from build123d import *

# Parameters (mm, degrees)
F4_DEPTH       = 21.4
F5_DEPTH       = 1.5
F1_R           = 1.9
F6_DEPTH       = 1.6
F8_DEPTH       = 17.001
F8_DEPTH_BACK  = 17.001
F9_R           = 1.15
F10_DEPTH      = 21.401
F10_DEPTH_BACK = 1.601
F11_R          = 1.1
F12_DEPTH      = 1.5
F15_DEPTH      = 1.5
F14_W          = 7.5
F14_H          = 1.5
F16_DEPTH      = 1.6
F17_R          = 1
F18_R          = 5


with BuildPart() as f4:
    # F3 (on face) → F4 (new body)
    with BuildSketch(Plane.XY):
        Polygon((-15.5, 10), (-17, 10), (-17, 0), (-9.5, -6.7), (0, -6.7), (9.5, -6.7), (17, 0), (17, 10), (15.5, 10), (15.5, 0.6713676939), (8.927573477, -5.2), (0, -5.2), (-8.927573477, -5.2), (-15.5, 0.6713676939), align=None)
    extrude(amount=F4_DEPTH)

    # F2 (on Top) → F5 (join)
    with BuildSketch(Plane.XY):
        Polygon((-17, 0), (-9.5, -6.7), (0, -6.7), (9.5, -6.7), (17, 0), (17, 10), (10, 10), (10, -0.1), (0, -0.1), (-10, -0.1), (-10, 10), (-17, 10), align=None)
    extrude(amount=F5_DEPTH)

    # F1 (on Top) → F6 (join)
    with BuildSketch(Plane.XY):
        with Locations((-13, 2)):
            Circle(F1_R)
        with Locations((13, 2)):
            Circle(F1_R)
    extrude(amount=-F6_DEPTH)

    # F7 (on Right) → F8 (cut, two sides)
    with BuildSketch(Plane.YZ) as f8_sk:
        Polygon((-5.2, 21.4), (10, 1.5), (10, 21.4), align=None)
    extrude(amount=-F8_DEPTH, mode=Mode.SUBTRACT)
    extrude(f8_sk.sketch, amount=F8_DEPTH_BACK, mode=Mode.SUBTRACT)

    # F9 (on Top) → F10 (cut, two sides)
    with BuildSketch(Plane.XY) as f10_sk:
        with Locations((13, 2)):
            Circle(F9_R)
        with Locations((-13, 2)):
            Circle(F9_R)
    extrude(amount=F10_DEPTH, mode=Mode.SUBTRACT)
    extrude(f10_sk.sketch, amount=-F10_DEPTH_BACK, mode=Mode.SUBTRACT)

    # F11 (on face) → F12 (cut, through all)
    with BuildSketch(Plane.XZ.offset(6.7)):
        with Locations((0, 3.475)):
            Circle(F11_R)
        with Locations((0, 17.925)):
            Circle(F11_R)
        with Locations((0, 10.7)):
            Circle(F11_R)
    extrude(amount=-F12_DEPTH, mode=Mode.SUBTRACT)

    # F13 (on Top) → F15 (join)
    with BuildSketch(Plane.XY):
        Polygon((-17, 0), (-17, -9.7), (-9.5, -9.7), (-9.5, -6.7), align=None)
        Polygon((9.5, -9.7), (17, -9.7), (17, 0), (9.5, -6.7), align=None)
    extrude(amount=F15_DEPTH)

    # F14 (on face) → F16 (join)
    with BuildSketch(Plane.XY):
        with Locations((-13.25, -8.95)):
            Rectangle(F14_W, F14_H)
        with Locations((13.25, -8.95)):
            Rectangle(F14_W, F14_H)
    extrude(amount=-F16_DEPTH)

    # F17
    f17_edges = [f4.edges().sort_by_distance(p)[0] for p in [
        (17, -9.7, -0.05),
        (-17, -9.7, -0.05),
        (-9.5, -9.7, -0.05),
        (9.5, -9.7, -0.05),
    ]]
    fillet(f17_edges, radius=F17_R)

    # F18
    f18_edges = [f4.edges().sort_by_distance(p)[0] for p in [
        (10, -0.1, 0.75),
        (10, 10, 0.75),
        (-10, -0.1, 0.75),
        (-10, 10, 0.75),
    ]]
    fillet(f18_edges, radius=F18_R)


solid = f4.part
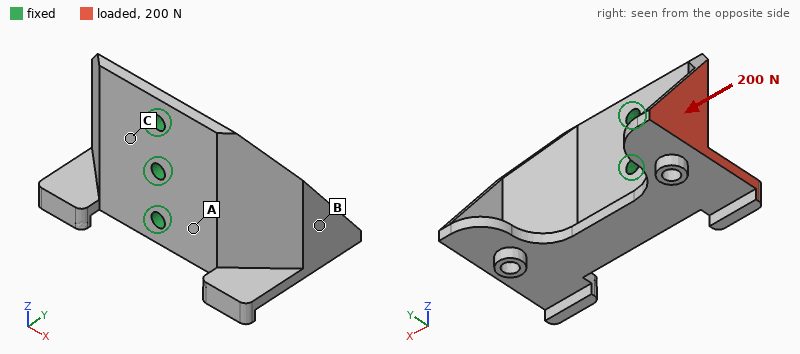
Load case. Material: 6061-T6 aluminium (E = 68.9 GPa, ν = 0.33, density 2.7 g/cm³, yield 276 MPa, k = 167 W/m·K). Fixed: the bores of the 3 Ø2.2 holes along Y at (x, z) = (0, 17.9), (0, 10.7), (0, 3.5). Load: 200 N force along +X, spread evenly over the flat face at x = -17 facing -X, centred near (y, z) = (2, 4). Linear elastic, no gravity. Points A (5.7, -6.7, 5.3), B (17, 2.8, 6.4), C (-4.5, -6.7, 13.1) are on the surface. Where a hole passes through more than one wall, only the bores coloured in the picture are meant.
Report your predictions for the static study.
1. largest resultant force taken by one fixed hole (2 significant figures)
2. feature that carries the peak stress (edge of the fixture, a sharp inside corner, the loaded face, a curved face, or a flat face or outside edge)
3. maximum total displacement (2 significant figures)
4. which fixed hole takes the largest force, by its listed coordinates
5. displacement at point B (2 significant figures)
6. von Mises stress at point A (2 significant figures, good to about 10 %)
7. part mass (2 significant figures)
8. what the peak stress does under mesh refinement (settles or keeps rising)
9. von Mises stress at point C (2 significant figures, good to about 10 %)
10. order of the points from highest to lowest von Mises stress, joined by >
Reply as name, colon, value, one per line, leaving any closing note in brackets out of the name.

largest resultant force taken by one fixed hole: 170 N
feature that carries the peak stress: edge of the fixture
maximum total displacement: 0.22 mm
which fixed hole takes the largest force, by its listed coordinates: (0, 3.5)
displacement at point B: 0.099 mm
von Mises stress at point A: 30 MPa
part mass: 5.0 g
what the peak stress does under mesh refinement: keeps rising
von Mises stress at point C: 51 MPa
order of the points from highest to lowest von Mises stress, joined by >: C > A > B
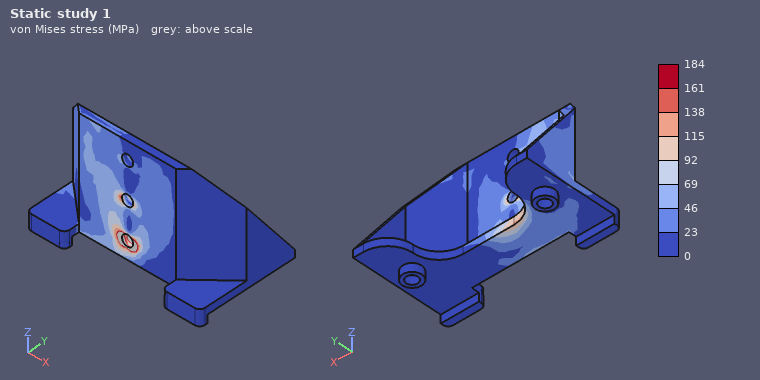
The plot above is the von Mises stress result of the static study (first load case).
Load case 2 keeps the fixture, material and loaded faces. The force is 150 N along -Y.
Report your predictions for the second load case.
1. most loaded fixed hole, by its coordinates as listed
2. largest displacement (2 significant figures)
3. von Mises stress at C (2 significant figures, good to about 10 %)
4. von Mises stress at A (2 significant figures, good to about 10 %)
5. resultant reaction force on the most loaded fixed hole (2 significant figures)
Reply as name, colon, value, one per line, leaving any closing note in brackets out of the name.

most loaded fixed hole, by its coordinates as listed: (0, 3.5)
largest displacement: 0.28 mm
von Mises stress at C: 75 MPa
von Mises stress at A: 38 MPa
resultant reaction force on the most loaded fixed hole: 130 N
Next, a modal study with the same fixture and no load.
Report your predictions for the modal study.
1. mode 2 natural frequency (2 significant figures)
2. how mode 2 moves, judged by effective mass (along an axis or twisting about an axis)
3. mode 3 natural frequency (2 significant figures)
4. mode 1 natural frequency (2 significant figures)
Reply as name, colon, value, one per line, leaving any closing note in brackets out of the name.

mode 2 natural frequency: 5800 Hz
how mode 2 moves, judged by effective mass: along Y
mode 3 natural frequency: 6100 Hz
mode 1 natural frequency: 3100 Hz
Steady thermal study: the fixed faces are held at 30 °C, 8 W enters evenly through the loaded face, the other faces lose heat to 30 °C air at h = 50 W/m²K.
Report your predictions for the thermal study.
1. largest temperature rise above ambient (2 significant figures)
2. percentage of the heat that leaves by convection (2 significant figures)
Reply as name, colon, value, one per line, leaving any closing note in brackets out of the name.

largest temperature rise above ambient: 28 K
percentage of the heat that leaves by convection: 11 %
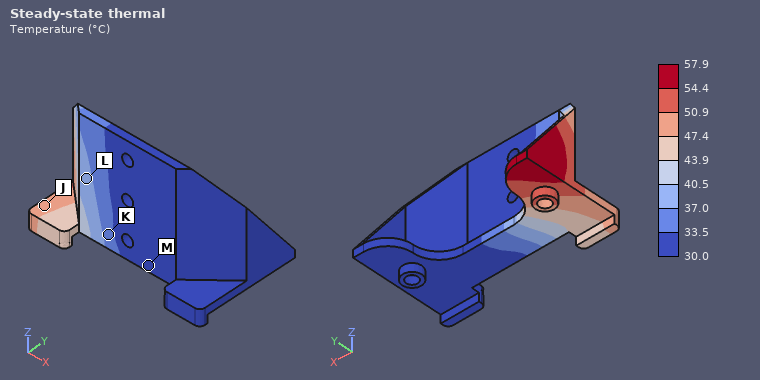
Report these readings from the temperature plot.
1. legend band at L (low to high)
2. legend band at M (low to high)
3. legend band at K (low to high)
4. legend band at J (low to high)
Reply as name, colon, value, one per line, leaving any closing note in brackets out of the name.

legend band at L: 37.0 to 40.5 °C
legend band at M: 30.0 to 33.5 °C
legend band at K: 33.5 to 37.0 °C
legend band at J: 47.4 to 50.9 °C
